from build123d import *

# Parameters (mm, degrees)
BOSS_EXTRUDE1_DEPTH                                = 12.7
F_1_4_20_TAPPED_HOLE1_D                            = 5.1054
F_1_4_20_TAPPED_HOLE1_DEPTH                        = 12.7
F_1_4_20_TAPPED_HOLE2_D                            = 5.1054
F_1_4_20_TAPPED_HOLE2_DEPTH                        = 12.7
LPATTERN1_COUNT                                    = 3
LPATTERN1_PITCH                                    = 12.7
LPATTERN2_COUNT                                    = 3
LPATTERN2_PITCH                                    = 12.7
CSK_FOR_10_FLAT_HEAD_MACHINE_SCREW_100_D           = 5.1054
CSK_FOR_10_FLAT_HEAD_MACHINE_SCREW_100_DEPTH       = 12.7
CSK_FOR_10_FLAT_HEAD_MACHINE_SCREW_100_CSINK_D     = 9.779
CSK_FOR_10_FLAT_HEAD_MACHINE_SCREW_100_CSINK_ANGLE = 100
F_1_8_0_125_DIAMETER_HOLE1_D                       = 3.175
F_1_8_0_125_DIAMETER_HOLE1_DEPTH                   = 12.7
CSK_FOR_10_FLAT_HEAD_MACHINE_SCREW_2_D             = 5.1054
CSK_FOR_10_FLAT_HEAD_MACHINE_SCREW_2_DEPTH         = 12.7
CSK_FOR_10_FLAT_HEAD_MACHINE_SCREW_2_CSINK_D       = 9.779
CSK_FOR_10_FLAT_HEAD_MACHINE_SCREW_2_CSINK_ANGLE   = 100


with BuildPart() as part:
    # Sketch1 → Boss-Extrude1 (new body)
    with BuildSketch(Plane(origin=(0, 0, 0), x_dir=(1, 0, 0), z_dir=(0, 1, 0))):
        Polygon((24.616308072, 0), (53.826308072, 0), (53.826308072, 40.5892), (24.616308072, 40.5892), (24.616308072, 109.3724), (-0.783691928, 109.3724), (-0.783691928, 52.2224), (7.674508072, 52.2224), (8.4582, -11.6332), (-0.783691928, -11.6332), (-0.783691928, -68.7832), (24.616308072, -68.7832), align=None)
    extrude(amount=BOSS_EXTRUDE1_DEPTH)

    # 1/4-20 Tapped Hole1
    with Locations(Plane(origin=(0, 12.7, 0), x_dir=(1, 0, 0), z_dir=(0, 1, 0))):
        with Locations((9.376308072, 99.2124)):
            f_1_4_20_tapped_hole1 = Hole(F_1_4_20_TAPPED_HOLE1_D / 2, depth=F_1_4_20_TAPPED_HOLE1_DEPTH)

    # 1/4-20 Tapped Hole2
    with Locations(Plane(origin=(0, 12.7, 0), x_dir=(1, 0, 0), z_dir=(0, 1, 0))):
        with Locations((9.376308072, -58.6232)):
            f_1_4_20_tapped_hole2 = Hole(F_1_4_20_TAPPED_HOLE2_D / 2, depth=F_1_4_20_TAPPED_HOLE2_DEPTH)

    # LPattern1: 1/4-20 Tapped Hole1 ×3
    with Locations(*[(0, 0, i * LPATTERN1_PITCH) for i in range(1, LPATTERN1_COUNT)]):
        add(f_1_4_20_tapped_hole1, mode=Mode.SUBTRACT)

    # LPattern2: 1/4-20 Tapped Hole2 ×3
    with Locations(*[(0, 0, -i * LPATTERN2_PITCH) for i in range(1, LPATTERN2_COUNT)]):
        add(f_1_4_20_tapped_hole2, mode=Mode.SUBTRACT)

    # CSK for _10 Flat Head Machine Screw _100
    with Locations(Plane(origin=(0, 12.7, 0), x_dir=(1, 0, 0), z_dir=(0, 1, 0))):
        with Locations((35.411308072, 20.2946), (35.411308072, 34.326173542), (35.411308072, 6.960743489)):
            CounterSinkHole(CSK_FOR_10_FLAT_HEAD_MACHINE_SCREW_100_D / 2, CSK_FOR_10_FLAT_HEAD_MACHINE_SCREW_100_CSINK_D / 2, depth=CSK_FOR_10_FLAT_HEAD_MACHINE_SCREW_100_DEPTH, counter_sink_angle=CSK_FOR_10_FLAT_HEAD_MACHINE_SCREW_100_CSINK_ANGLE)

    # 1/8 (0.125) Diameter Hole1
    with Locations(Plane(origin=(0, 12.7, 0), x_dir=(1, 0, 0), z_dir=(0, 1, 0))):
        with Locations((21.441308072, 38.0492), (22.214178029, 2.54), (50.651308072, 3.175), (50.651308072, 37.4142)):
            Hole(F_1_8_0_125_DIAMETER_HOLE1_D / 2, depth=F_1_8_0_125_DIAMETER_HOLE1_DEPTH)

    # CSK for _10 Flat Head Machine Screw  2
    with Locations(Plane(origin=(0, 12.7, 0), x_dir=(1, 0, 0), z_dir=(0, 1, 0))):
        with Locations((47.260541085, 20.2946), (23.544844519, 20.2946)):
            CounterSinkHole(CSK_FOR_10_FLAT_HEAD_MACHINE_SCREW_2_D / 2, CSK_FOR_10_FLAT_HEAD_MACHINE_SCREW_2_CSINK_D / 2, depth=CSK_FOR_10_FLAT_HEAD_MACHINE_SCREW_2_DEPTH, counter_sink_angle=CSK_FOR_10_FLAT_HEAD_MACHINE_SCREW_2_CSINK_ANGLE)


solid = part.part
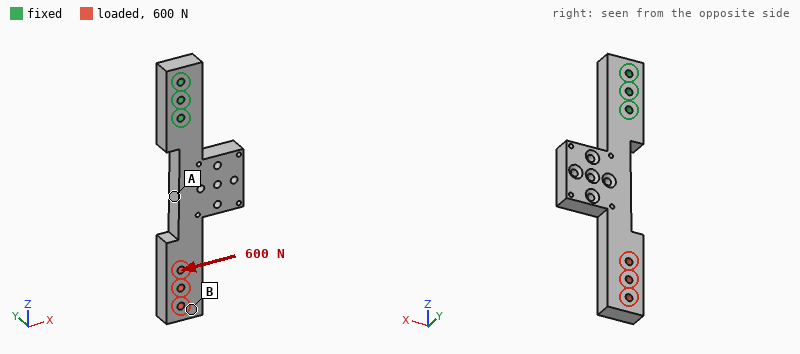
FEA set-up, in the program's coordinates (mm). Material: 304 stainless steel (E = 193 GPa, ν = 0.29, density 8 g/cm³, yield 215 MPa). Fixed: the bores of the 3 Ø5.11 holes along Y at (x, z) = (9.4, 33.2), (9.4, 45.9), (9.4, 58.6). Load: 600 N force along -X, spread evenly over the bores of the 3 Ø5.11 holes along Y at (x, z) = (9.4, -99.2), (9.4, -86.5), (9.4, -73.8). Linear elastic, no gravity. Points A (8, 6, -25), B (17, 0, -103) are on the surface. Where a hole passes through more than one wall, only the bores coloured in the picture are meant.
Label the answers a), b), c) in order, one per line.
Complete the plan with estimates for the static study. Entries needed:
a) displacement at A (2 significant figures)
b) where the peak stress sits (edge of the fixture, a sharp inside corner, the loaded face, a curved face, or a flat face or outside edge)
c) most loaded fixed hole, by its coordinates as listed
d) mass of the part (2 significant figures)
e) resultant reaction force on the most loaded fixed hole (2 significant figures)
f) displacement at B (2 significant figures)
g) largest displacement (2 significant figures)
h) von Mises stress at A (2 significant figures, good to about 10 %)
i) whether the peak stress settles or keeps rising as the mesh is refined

a) 0.082 mm
b) a sharp inside corner
c) (9.4, 33.2)
d) 490 g
e) 3.5 kN
f) 0.31 mm
g) 0.33 mm
h) 25 MPa
i) keeps rising
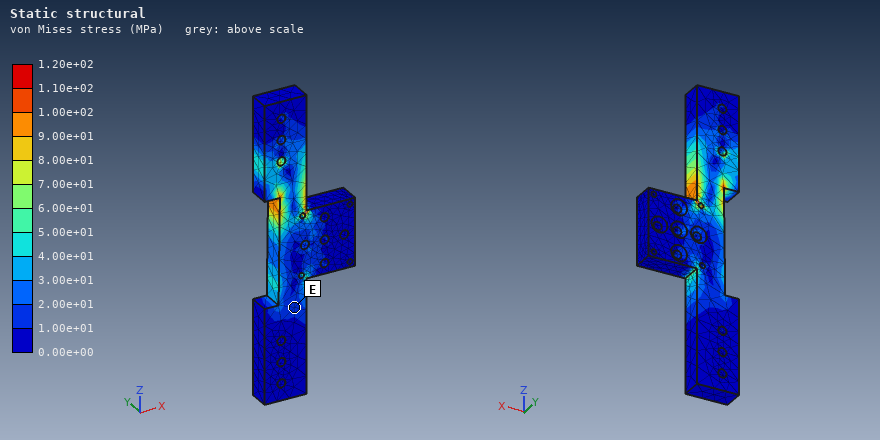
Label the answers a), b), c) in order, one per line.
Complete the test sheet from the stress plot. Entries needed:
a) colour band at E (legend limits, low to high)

a) 1.00e+01 to 2.00e+01 MPa
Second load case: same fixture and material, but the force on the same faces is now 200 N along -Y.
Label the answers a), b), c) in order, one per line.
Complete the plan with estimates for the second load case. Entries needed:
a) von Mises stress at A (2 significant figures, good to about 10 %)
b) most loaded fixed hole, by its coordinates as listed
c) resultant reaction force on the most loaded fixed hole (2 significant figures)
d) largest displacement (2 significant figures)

a) 5.6 MPa
b) (9.4, 33.2)
c) 680 N
d) 0.24 mm
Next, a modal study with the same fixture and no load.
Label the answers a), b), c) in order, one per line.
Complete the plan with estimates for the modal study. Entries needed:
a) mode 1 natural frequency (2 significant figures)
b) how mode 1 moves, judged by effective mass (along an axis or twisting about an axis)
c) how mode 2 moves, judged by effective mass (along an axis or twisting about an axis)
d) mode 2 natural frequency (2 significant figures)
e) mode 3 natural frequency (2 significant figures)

a) 430 Hz
b) along Y
c) along X
d) 620 Hz
e) 1600 Hz
